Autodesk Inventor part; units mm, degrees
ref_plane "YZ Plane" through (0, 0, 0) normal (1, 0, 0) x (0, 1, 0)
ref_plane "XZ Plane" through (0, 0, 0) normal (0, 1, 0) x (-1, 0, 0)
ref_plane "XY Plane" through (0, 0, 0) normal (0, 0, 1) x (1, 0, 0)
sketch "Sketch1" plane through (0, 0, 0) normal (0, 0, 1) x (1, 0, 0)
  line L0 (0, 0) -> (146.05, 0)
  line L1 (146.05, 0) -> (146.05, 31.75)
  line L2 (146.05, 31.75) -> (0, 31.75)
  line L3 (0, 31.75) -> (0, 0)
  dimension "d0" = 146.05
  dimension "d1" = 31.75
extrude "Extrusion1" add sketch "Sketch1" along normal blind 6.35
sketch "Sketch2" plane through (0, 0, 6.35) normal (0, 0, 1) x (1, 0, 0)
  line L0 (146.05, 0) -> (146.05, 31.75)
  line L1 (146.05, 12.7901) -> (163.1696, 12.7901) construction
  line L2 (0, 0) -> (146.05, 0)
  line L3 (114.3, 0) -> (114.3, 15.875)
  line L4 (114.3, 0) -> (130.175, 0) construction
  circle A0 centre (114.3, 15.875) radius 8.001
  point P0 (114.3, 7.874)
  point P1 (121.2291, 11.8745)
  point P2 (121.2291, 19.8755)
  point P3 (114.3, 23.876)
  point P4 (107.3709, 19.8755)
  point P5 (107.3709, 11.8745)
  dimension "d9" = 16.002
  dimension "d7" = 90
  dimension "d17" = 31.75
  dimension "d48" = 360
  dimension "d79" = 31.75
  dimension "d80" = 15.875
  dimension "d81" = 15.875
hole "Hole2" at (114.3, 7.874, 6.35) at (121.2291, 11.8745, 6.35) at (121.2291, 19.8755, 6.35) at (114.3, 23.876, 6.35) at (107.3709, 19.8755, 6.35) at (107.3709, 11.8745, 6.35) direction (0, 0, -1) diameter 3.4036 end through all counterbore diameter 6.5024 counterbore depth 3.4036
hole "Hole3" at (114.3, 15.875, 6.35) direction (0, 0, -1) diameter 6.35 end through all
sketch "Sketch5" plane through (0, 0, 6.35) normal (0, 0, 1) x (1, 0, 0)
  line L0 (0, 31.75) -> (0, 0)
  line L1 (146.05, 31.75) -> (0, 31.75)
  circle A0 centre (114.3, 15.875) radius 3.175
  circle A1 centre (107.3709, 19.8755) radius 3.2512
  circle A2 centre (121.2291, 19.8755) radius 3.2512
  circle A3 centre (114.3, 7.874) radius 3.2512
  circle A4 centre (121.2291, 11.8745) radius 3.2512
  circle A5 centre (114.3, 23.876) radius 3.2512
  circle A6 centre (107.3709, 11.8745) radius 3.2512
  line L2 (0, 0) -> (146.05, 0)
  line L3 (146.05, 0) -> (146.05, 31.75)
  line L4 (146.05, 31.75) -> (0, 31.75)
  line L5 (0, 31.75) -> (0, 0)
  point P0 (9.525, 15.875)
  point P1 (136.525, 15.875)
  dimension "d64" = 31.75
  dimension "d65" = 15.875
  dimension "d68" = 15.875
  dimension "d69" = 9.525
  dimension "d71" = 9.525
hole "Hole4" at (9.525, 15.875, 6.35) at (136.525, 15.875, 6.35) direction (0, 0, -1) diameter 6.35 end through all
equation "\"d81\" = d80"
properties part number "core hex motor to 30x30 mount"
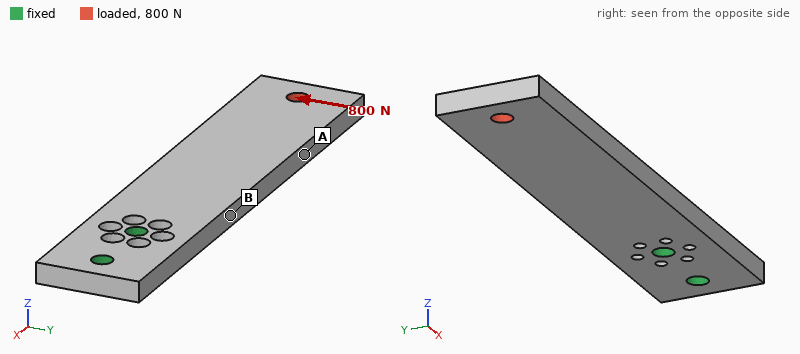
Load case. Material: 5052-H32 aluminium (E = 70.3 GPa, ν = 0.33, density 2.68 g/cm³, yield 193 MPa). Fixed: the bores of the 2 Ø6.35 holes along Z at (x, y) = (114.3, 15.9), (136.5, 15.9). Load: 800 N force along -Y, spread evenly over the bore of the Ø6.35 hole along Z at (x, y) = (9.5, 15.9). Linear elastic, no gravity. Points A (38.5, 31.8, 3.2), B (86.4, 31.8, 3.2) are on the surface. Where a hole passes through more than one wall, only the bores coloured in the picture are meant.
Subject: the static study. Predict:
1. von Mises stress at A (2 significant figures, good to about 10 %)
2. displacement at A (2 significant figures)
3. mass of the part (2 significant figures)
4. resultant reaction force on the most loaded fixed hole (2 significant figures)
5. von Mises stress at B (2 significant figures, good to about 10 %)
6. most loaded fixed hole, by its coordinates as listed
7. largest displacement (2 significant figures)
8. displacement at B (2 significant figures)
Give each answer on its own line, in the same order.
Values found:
22 MPa
0.29 mm
75 g
3.4 kN
58 MPa
(114.3, 15.9)
0.49 mm
0.090 mm
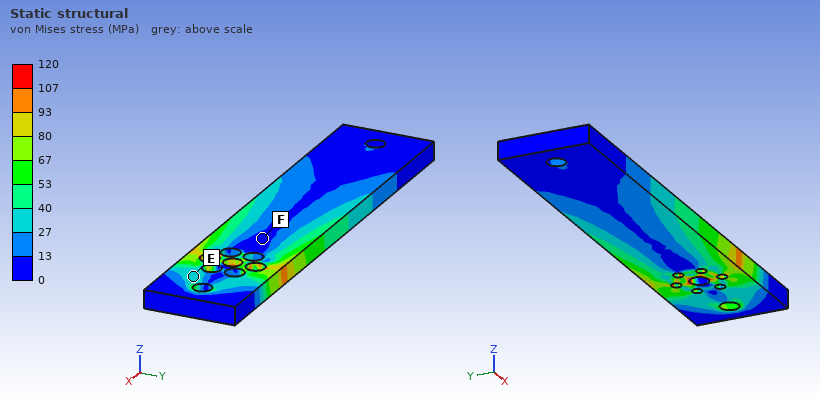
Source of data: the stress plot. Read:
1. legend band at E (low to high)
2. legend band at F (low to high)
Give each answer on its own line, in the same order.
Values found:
27 to 40 MPa
0 to 13 MPa
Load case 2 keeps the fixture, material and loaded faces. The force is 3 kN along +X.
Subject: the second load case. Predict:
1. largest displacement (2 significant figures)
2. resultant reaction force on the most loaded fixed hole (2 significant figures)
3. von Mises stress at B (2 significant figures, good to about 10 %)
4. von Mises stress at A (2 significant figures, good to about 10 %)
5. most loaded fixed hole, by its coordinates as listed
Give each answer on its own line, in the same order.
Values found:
74 µm
2.2 kN
15 MPa
15 MPa
(114.3, 15.9)
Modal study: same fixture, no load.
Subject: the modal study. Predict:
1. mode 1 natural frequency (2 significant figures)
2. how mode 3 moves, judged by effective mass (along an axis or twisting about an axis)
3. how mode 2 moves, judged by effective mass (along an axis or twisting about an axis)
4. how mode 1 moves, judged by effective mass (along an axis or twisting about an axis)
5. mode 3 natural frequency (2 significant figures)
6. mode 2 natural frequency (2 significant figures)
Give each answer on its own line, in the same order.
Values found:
370 Hz
along Z
along Y
along Z
2300 Hz
1500 Hz
